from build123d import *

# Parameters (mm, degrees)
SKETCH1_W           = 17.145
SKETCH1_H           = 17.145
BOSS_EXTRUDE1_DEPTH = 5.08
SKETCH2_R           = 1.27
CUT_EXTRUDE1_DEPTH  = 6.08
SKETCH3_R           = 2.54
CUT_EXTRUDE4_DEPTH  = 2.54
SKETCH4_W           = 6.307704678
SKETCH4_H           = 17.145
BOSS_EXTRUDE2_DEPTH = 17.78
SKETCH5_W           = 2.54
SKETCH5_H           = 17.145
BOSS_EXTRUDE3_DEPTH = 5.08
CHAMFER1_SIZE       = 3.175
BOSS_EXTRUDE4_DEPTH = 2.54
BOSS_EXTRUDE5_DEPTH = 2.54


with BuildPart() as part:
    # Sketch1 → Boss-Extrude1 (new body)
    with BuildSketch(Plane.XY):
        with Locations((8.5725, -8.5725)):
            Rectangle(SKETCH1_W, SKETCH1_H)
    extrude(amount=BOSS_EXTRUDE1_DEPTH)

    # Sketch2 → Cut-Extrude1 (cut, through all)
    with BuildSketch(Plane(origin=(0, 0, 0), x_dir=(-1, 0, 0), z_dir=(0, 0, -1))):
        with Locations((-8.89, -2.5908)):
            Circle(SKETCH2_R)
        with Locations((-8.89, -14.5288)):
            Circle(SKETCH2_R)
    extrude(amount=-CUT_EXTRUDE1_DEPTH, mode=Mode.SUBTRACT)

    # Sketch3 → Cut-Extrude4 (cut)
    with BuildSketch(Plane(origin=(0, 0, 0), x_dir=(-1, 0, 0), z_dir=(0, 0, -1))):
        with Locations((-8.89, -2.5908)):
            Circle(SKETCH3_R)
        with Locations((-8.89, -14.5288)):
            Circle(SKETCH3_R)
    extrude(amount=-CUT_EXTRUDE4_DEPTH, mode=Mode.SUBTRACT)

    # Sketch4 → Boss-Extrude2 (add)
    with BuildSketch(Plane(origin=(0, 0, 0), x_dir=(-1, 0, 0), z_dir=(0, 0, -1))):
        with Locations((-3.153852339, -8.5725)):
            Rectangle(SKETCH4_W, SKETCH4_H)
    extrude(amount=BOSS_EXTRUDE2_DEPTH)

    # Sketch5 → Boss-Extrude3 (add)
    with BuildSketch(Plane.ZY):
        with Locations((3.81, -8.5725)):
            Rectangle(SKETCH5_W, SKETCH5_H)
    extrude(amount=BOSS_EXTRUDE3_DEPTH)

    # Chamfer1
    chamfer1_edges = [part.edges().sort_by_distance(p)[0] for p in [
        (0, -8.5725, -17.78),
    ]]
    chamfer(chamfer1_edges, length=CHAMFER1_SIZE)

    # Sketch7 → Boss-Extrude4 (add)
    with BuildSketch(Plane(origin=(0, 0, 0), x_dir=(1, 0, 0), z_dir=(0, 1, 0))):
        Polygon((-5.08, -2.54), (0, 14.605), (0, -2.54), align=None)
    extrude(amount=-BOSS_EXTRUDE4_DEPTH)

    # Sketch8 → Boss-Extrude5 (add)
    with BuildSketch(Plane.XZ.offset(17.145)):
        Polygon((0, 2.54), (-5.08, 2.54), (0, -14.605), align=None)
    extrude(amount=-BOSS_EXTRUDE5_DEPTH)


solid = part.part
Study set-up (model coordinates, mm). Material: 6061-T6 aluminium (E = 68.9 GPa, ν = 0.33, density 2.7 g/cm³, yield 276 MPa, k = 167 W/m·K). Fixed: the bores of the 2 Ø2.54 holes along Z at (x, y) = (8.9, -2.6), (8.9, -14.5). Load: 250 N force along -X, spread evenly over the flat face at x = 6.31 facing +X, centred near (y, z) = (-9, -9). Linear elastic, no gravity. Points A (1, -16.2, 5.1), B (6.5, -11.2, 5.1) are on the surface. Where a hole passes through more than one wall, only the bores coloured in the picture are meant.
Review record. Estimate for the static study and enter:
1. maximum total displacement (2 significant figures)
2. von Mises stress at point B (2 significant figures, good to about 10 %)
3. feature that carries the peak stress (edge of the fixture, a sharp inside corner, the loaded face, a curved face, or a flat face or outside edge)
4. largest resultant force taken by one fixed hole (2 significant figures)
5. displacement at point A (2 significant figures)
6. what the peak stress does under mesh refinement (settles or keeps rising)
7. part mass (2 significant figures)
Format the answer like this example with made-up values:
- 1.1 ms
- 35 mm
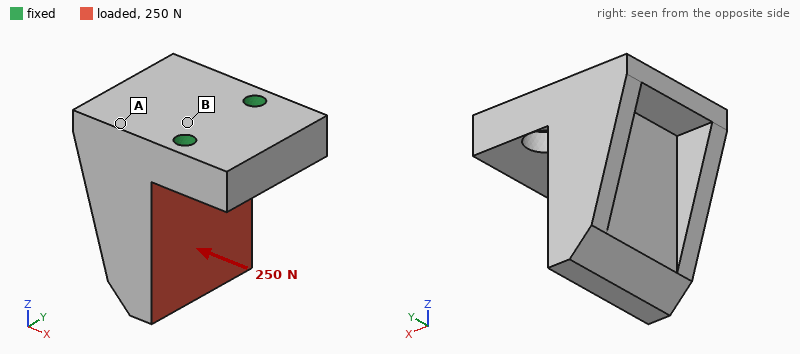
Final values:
- 73 µm
- 41 MPa
- edge of the fixture
- 130 N
- 20 µm
- keeps rising
- 9.8 g
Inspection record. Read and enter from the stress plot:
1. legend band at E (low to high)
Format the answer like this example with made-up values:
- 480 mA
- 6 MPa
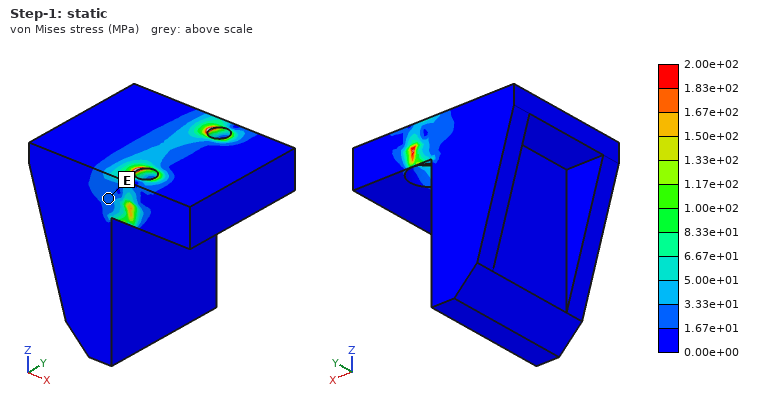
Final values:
- 1.67e+01 to 3.33e+01 MPa
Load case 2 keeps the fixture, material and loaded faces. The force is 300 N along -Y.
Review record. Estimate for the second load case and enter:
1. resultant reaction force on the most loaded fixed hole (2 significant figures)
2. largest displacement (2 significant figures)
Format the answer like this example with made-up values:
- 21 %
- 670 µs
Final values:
- 340 N
- 19 µm
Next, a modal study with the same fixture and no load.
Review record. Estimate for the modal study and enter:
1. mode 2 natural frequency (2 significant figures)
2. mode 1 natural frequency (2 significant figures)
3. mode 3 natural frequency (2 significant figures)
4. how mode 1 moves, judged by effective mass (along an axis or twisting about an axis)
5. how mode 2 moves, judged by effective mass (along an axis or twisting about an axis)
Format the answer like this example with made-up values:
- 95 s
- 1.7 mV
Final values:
- 11 kHz
- 4600 Hz
- 21 kHz
- along X
- along Y
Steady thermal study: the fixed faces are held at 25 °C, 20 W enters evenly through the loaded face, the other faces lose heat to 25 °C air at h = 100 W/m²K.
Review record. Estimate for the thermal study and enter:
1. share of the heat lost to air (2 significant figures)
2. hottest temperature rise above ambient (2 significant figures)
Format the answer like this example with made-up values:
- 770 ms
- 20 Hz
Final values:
- 8.9 %
- 20 K
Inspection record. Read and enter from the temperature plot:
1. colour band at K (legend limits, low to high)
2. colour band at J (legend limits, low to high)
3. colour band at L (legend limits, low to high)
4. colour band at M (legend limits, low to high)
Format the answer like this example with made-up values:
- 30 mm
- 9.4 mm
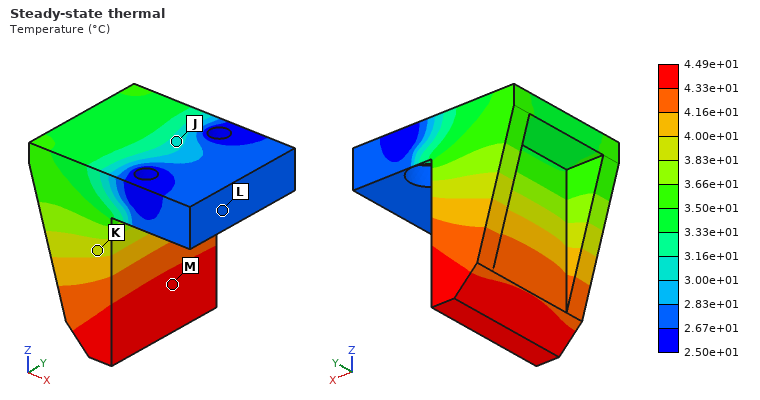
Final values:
- 3.83e+01 to 4.00e+01 °C
- 3.00e+01 to 3.16e+01 °C
- 2.67e+01 to 2.83e+01 °C
- 4.33e+01 to 4.49e+01 °C
